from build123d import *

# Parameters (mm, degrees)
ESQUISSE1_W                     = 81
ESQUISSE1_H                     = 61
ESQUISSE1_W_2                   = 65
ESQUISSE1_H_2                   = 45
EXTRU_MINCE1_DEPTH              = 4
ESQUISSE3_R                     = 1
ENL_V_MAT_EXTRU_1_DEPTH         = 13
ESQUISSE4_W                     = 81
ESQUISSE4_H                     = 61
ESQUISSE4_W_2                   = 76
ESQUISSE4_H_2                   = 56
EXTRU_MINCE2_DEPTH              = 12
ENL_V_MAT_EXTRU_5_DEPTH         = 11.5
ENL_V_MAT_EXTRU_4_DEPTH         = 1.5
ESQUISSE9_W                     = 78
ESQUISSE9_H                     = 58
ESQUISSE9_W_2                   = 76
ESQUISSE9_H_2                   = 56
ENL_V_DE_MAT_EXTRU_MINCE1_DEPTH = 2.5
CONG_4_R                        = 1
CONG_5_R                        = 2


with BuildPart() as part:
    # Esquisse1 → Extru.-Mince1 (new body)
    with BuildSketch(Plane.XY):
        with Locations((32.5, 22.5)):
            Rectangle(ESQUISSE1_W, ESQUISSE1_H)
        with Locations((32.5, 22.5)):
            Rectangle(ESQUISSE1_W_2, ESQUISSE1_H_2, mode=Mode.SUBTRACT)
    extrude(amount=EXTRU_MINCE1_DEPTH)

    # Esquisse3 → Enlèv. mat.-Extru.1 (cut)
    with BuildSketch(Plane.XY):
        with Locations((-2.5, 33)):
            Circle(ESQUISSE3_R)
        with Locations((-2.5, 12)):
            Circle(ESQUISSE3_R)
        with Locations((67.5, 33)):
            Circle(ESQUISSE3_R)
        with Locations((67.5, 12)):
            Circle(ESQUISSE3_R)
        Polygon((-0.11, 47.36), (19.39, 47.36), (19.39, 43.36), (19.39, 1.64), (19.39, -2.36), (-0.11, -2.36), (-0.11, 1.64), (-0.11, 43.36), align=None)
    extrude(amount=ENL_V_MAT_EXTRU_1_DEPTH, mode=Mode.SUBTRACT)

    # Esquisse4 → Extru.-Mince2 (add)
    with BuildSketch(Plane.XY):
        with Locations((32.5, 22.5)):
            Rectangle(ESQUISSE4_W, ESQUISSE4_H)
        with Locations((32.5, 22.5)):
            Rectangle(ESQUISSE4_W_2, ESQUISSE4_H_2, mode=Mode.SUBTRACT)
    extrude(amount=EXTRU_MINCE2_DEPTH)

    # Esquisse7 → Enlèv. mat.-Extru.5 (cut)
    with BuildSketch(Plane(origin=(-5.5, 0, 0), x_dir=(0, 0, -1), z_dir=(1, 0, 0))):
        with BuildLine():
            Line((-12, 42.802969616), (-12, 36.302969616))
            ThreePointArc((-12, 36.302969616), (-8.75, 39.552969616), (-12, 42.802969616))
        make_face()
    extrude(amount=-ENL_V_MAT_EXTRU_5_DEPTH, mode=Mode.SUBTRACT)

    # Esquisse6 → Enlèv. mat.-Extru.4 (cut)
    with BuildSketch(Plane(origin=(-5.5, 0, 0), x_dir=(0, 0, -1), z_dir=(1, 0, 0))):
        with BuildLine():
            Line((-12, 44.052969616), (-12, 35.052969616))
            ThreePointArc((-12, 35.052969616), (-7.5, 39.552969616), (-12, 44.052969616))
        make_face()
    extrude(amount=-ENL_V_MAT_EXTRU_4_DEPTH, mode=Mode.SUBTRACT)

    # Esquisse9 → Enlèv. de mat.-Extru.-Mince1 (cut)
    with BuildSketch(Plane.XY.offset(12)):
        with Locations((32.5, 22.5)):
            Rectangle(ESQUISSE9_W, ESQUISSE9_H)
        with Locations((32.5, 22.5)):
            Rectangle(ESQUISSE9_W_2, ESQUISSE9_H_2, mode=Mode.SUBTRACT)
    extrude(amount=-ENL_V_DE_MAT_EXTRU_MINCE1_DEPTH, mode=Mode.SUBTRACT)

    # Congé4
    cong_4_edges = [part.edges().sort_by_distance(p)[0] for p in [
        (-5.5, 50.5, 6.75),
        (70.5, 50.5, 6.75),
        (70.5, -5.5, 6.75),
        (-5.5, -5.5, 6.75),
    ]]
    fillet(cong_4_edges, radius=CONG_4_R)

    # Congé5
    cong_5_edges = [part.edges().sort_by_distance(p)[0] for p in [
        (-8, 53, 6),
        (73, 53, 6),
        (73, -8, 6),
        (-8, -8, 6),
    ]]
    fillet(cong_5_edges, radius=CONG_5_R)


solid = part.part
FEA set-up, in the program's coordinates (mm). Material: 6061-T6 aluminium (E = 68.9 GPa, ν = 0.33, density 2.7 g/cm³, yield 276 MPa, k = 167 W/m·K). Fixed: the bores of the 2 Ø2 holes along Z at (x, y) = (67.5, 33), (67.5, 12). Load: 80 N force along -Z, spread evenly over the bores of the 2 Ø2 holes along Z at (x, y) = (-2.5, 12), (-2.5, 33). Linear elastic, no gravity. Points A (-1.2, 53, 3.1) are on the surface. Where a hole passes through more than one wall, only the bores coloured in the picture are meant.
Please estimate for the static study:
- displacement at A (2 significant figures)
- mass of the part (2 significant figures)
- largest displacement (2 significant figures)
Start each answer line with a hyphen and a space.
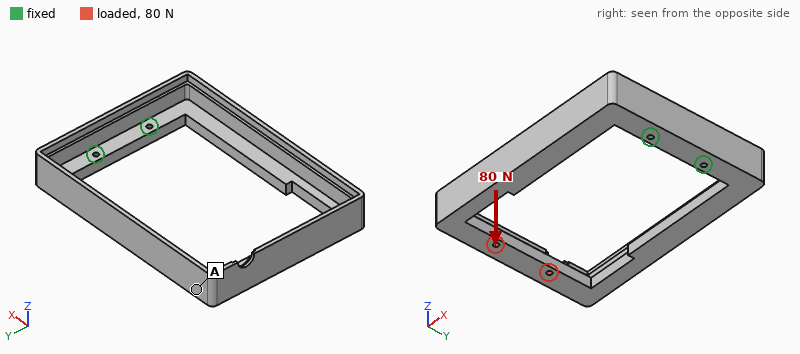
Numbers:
- 0.96 mm
- 33 g
- 1.1 mm
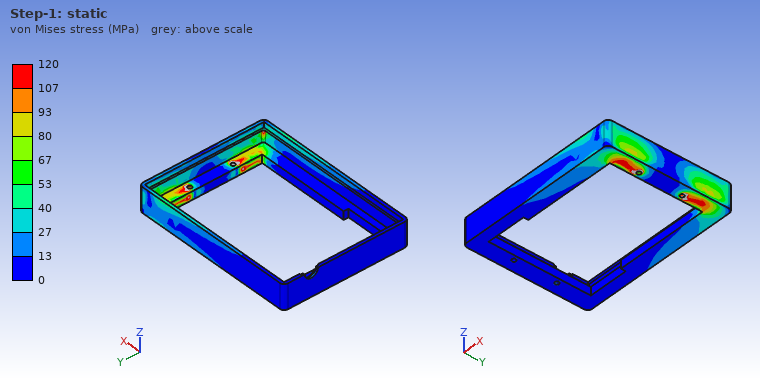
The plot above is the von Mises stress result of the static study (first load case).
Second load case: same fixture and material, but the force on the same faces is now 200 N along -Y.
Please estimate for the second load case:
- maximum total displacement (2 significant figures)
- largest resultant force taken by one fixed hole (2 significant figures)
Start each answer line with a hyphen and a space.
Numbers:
- 0.88 mm
- 490 N
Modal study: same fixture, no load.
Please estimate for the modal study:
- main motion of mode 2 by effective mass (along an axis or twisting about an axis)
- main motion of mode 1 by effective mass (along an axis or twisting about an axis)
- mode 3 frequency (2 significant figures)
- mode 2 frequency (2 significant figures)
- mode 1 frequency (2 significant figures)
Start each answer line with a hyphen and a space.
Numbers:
- along Y
- along Z
- 880 Hz
- 640 Hz
- 390 Hz
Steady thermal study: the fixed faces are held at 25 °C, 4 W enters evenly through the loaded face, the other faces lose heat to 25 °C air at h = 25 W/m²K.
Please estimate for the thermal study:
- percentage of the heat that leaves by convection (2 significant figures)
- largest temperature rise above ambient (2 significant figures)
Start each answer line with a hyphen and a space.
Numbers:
- 49 %
- 18 K
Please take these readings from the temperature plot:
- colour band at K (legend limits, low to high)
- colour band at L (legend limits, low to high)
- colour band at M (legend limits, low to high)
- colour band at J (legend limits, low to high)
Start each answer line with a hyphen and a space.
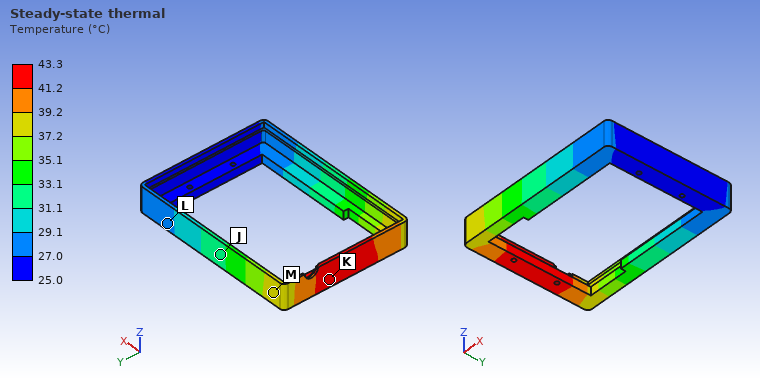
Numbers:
- 41.2 to 43.3 °C
- 27.0 to 29.1 °C
- 37.2 to 39.2 °C
- 31.1 to 33.1 °C
